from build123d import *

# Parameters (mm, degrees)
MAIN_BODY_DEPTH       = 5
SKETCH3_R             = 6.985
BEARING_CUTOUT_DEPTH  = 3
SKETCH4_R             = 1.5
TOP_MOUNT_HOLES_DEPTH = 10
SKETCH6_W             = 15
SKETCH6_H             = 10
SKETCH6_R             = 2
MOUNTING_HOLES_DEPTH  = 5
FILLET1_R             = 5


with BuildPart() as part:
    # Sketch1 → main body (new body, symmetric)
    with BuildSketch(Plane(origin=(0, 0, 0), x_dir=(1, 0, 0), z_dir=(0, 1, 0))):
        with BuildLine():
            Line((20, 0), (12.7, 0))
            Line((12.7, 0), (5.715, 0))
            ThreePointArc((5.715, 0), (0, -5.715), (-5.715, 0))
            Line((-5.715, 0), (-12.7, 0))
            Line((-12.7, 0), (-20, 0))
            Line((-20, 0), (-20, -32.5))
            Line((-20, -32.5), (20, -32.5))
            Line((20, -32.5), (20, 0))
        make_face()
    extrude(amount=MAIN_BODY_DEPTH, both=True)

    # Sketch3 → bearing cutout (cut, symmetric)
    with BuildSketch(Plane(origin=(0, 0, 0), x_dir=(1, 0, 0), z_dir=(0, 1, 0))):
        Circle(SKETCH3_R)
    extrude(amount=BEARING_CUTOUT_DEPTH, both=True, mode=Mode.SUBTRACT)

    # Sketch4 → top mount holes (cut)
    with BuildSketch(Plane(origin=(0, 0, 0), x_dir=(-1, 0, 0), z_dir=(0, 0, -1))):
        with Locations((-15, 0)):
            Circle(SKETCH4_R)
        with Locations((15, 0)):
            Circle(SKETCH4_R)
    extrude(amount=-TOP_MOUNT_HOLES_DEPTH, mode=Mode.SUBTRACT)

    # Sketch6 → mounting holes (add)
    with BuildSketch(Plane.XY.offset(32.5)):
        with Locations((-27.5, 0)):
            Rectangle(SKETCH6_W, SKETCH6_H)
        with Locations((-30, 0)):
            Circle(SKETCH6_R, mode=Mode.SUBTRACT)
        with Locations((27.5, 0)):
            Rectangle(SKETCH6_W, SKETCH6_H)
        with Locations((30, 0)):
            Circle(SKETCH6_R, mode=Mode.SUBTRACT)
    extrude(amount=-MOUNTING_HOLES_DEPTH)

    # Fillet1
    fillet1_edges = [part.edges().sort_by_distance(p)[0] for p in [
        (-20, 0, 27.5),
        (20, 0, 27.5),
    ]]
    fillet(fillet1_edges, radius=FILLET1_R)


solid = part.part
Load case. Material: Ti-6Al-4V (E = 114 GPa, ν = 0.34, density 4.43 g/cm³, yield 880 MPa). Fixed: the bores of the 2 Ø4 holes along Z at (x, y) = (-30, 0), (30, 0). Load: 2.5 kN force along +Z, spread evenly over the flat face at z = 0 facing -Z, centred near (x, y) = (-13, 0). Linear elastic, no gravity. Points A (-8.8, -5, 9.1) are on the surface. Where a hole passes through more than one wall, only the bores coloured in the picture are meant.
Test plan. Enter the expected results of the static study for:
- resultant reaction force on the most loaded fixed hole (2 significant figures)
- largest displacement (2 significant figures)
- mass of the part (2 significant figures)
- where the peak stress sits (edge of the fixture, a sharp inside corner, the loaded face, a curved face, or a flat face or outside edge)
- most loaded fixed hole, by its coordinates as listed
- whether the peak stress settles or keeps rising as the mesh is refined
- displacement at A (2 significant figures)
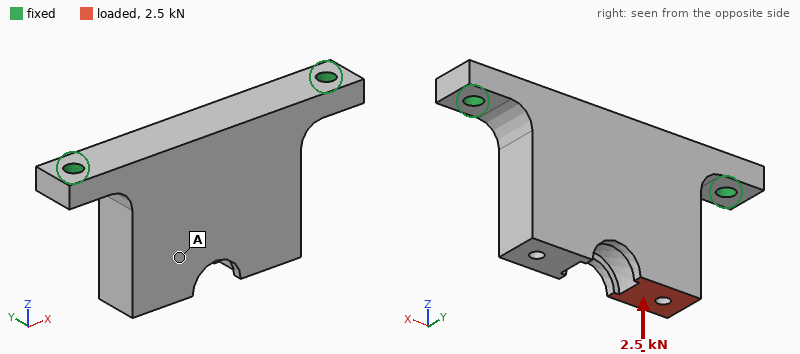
2.1 kN
29 µm
61 g
edge of the fixture
(-30, 0)
keeps rising
21 µm
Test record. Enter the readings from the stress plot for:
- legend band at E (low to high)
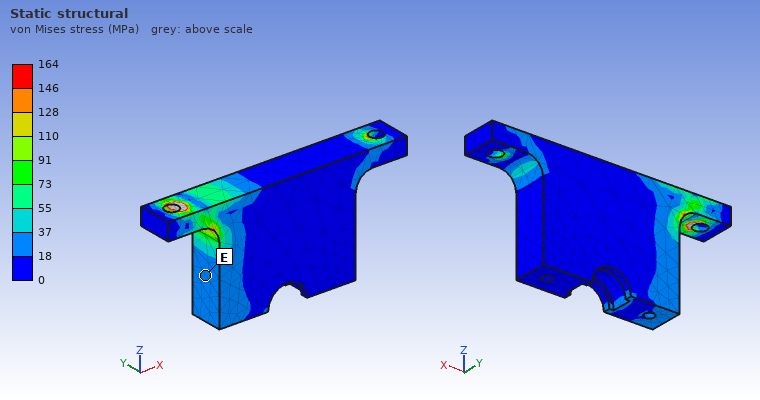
18 to 37 MPa
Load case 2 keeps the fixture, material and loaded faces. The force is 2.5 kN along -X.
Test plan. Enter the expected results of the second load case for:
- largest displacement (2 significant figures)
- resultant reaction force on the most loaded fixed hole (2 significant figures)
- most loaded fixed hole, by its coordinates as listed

42 µm
2.1 kN
(30, 0)
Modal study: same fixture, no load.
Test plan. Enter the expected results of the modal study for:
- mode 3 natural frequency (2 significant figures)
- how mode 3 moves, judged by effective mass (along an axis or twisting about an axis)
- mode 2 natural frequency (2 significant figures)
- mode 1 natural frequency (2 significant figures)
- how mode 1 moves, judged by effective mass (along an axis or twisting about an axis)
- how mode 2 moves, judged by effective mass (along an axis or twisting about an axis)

10 kHz
twisting about Z
8400 Hz
2300 Hz
along Y
along Z
